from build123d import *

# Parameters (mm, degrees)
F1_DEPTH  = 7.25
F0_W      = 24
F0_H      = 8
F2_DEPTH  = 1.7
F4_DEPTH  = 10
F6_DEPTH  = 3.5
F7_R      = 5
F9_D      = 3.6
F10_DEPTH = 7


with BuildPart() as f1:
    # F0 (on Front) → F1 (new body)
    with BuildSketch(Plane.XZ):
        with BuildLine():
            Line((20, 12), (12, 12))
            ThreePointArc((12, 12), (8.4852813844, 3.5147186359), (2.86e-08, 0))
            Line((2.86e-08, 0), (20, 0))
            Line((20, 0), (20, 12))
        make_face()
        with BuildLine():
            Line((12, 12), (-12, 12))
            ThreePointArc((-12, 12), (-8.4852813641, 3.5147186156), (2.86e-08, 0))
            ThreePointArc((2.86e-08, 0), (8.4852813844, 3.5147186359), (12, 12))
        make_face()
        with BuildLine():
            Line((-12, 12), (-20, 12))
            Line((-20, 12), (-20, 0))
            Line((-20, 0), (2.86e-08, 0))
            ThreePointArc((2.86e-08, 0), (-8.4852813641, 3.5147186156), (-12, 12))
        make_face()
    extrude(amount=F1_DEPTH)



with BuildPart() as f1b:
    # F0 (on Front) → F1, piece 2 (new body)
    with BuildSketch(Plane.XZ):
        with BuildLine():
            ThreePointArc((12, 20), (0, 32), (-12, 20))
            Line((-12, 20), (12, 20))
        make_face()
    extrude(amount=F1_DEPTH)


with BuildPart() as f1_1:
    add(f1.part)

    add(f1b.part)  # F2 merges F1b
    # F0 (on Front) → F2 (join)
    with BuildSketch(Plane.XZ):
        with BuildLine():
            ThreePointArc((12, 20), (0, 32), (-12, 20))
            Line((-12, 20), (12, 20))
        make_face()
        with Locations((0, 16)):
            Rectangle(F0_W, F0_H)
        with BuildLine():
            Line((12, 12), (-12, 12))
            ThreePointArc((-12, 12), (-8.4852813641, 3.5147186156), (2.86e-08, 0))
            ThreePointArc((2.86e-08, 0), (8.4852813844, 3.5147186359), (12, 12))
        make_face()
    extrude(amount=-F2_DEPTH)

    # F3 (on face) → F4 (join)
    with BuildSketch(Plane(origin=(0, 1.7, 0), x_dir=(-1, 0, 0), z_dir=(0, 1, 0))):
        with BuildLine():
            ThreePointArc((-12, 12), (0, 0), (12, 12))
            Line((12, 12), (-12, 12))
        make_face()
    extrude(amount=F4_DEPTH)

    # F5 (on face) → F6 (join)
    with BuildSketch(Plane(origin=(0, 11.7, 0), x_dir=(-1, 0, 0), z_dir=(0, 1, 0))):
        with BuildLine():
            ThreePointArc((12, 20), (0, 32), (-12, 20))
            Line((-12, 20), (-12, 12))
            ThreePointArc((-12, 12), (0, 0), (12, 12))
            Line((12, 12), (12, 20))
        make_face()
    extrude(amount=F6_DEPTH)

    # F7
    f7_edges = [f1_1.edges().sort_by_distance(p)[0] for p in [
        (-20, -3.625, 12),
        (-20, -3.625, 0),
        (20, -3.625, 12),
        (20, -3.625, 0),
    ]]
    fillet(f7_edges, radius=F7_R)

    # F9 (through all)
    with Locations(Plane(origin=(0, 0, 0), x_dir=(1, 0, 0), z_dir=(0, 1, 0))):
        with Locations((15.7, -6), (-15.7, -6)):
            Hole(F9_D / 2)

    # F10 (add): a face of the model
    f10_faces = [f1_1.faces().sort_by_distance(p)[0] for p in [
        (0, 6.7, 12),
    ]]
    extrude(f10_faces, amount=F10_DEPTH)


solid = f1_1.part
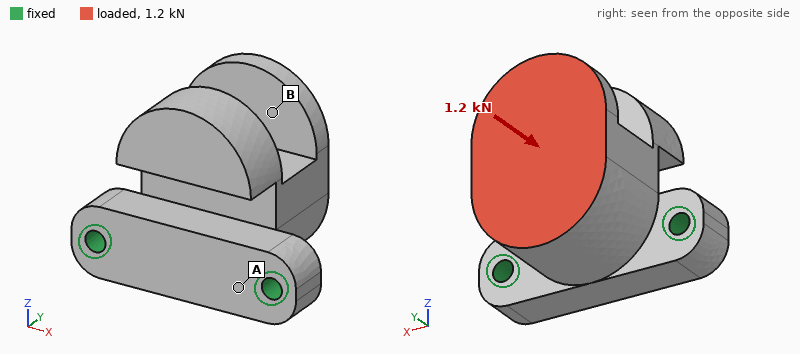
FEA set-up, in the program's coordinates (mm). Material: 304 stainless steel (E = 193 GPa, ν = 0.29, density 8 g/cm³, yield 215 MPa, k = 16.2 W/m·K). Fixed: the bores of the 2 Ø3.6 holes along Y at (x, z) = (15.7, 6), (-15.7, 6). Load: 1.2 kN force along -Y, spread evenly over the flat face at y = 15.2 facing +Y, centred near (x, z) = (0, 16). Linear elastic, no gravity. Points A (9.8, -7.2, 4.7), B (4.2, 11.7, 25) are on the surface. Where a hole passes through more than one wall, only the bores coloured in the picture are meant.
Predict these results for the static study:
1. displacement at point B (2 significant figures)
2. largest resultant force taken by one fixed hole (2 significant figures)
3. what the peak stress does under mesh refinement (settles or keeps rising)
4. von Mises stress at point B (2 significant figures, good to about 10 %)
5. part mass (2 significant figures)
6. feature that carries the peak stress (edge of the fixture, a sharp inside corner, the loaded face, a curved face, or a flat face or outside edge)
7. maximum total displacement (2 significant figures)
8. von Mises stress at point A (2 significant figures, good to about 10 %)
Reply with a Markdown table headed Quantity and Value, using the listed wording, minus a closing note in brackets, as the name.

| Quantity | Value |
|---|---|
| displacement at point B | 22 µm |
| largest resultant force taken by one fixed hole | 640 N |
| what the peak stress does under mesh refinement | keeps rising |
| von Mises stress at point B | 15 MPa |
| part mass | 97 g |
| feature that carries the peak stress | edge of the fixture |
| maximum total displacement | 36 µm |
| von Mises stress at point A | 36 MPa |
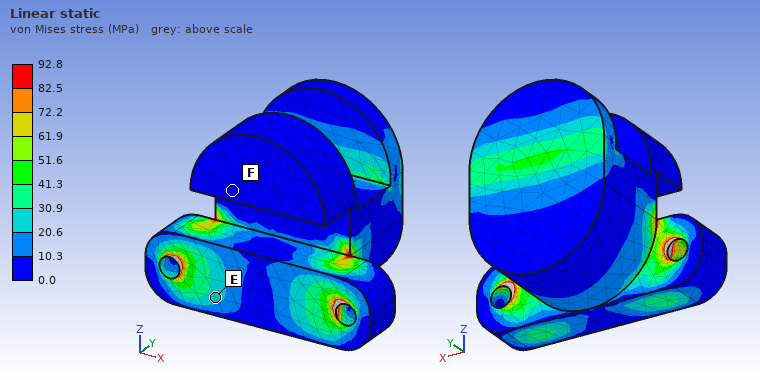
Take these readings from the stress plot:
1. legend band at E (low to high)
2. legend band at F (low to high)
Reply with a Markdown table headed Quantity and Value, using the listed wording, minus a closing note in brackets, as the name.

| Quantity | Value |
|---|---|
| legend band at E | 20.6 to 30.9 MPa |
| legend band at F | 0.0 to 10.3 MPa |
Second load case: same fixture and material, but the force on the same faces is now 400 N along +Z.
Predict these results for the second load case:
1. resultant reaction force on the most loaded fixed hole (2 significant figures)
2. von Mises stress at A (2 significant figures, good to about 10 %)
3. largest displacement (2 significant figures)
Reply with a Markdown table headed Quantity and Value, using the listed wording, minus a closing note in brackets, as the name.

| Quantity | Value |
|---|---|
| resultant reaction force on the most loaded fixed hole | 200 N |
| von Mises stress at A | 21 MPa |
| largest displacement | 17 µm |
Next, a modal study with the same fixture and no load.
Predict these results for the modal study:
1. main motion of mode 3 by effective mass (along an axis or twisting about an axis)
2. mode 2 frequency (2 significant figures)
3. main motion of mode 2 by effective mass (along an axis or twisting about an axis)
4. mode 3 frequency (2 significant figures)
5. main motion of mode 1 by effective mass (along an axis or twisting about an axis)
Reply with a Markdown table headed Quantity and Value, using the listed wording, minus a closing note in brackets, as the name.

| Quantity | Value |
|---|---|
| main motion of mode 3 by effective mass | along X |
| mode 2 frequency | 5700 Hz |
| main motion of mode 2 by effective mass | along Z |
| mode 3 frequency | 11 kHz |
| main motion of mode 1 by effective mass | along Y |
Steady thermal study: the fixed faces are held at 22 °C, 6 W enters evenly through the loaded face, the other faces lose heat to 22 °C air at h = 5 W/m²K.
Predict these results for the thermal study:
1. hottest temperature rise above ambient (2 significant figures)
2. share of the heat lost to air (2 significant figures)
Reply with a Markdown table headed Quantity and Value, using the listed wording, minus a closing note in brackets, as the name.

| Quantity | Value |
|---|---|
| hottest temperature rise above ambient | 50 K |
| share of the heat lost to air | 7.2 % |
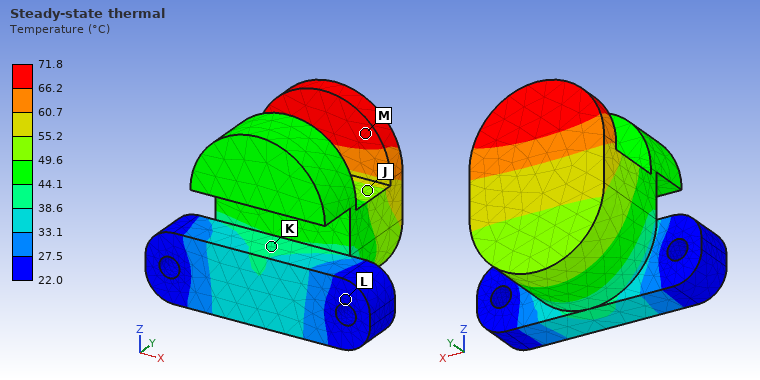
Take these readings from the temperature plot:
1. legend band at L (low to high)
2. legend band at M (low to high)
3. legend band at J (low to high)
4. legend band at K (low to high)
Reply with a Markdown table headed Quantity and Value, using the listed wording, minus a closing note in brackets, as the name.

| Quantity | Value |
|---|---|
| legend band at L | 22.0 to 27.5 °C |
| legend band at M | 66.2 to 71.8 °C |
| legend band at J | 49.6 to 55.2 °C |
| legend band at K | 38.6 to 44.1 °C |
